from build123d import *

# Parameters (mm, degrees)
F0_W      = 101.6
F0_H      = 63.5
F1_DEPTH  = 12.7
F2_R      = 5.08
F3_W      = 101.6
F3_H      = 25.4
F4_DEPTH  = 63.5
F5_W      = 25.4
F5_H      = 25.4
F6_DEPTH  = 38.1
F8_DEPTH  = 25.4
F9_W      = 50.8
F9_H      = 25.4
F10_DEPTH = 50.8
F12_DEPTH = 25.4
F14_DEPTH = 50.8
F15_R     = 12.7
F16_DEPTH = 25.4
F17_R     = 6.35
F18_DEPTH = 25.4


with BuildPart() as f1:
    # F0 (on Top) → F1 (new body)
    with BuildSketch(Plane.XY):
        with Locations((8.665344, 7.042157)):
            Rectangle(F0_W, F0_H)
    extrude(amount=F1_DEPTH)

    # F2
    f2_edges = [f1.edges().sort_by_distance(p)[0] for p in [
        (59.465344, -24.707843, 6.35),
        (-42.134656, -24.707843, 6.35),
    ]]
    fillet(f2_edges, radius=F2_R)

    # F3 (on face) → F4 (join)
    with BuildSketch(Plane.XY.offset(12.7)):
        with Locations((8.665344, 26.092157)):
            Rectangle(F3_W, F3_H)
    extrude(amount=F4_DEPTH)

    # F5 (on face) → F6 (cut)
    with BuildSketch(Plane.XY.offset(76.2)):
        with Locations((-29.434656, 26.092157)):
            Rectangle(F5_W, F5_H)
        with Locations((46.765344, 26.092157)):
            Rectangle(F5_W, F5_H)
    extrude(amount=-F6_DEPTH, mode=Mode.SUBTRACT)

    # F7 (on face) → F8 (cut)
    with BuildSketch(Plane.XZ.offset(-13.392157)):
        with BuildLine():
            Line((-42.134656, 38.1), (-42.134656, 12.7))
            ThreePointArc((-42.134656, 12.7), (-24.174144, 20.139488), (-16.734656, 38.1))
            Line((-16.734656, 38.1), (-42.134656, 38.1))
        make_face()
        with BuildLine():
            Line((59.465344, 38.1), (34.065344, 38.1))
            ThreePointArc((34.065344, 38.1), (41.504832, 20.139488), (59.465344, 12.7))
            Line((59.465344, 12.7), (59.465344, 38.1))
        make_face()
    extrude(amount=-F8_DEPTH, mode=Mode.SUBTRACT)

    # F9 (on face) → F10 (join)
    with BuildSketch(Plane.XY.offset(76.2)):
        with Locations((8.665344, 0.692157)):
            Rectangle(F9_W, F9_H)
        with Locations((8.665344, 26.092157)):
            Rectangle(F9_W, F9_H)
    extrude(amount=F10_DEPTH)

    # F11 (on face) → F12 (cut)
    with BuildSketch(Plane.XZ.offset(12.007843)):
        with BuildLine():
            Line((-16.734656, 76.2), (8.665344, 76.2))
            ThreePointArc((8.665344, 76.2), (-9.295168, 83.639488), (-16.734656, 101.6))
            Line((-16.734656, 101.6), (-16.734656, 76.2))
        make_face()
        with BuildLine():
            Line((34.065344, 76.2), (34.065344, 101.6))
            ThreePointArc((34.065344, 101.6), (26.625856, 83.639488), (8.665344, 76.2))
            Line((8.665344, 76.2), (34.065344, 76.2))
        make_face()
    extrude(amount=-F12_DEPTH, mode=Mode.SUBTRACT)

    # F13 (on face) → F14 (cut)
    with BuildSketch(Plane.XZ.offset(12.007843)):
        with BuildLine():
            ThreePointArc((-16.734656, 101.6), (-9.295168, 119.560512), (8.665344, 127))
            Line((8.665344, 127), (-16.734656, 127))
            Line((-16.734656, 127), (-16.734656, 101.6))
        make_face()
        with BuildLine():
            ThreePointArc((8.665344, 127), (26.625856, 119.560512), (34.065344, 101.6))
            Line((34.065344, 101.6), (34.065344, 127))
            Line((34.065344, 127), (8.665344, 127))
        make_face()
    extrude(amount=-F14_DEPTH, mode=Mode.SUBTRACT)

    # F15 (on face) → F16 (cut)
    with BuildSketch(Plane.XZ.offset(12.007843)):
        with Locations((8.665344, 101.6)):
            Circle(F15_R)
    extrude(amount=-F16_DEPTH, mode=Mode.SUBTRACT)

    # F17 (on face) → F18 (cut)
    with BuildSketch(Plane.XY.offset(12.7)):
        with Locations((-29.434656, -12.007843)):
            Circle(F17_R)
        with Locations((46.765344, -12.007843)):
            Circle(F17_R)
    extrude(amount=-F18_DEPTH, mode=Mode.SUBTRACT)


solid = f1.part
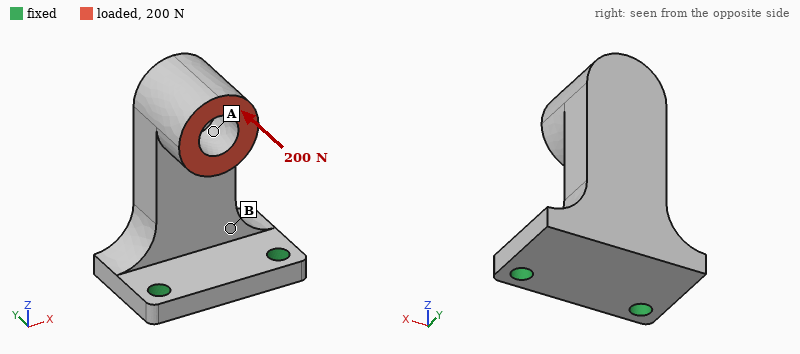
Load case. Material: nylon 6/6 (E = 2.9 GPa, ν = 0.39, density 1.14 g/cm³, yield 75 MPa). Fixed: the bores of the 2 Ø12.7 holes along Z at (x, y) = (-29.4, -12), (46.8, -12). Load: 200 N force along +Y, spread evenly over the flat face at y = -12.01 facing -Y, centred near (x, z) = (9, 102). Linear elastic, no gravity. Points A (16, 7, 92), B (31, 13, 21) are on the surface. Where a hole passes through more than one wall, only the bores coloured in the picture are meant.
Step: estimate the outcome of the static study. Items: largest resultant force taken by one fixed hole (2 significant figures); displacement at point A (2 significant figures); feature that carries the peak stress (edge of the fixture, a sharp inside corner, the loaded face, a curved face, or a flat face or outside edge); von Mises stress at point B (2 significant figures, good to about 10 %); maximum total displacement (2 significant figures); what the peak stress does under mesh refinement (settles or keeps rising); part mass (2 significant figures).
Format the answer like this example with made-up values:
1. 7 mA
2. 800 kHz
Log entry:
1. 120 N
2. 1.2 mm
3. edge of the fixture
4. 3.0 MPa
5. 1.8 mm
6. keeps rising
7. 300 g
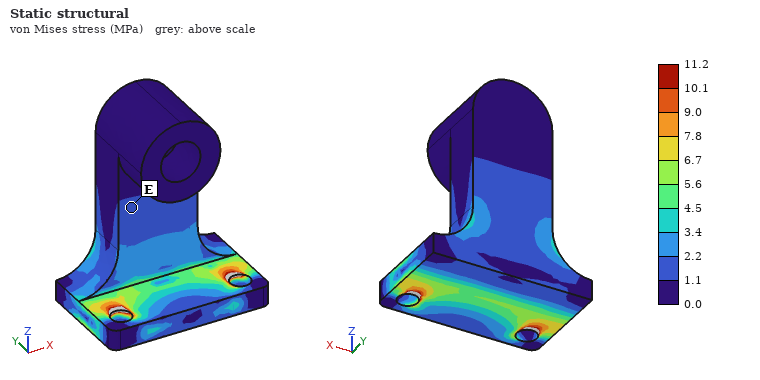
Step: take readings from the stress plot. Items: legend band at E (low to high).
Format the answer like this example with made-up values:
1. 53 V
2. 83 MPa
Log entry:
1. 1.1 to 2.2 MPa
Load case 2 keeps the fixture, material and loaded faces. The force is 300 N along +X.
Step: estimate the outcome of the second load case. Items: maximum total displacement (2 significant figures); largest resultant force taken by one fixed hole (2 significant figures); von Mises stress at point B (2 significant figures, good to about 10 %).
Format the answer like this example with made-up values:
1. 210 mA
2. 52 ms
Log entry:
1. 0.70 mm
2. 410 N
3. 3.6 MPa
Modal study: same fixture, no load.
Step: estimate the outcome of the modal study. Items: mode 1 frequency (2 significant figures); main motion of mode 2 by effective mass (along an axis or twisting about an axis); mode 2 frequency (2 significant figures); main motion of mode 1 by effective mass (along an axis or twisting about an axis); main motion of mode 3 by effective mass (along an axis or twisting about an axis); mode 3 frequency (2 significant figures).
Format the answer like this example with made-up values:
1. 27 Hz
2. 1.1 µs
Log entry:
1. 160 Hz
2. along X
3. 390 Hz
4. along Y
5. along Z
6. 760 Hz
